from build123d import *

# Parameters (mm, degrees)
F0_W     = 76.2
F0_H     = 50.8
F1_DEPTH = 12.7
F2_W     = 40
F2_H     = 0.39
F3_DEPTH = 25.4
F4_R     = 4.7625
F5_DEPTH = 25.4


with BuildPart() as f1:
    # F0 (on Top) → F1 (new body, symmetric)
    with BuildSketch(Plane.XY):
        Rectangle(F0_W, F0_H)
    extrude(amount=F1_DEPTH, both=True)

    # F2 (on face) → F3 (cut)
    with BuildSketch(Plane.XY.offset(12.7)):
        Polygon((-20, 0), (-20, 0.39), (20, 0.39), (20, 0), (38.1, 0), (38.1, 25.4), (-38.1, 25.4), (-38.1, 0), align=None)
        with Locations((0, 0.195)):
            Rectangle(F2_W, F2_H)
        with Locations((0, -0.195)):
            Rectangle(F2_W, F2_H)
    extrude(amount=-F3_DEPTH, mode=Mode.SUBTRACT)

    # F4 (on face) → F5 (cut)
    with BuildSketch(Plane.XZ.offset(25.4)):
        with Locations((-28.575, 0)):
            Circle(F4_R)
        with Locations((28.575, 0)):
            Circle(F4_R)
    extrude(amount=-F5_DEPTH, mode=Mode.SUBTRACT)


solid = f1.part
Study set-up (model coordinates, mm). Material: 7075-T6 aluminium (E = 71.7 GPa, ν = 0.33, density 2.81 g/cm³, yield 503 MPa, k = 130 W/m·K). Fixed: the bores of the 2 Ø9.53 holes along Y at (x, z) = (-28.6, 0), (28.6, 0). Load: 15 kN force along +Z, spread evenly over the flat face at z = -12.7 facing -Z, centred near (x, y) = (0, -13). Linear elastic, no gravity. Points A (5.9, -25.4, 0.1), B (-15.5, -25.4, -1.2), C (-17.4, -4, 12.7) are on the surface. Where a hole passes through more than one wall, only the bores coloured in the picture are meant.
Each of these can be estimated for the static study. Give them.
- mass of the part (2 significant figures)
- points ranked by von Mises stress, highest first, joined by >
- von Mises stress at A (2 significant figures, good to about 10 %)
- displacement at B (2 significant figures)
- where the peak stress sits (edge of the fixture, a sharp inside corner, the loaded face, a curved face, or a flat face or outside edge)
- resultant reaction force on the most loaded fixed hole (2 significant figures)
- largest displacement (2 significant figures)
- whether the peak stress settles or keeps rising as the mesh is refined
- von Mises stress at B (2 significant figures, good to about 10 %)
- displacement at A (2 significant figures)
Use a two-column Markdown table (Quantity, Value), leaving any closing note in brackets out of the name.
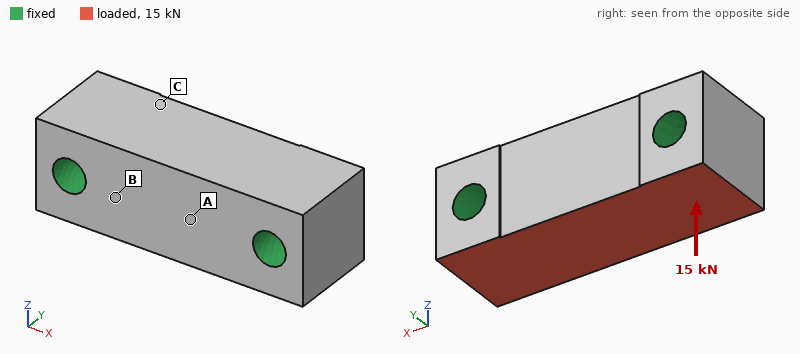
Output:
| Quantity | Value |
|---|---|
| mass of the part | 130 g |
| points ranked by von Mises stress, highest first, joined by > | B > A > C |
| von Mises stress at A | 6.3 MPa |
| displacement at B | 4.6 µm |
| where the peak stress sits | edge of the fixture |
| resultant reaction force on the most loaded fixed hole | 7.5 kN |
| largest displacement | 8.6 µm |
| whether the peak stress settles or keeps rising as the mesh is refined | keeps rising |
| von Mises stress at B | 13 MPa |
| displacement at A | 7.3 µm |
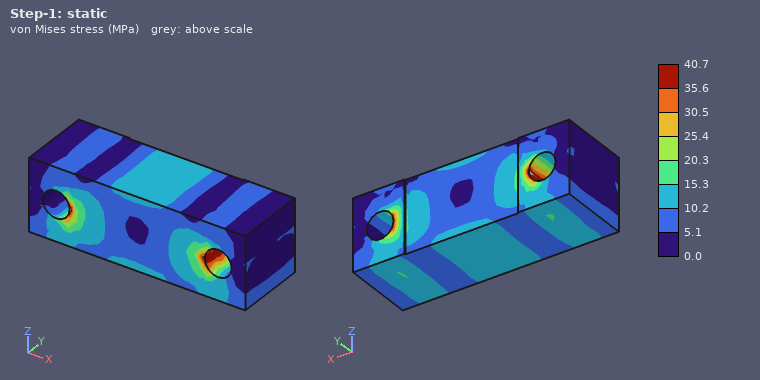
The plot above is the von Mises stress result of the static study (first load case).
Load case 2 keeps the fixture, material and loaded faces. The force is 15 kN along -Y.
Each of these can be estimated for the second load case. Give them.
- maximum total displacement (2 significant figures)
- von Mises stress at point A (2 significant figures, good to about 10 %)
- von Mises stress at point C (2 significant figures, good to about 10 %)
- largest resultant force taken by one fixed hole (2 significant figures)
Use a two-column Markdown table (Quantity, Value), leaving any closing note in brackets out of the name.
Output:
| Quantity | Value |
|---|---|
| maximum total displacement | 20 µm |
| von Mises stress at point A | 14 MPa |
| von Mises stress at point C | 7.8 MPa |
| largest resultant force taken by one fixed hole | 7.5 kN |
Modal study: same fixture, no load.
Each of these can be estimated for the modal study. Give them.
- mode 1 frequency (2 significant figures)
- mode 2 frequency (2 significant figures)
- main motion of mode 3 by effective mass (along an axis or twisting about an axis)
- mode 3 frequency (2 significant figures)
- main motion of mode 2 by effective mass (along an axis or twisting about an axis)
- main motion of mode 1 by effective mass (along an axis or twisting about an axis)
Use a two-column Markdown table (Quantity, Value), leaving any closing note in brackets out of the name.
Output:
| Quantity | Value |
|---|---|
| mode 1 frequency | 21 kHz |
| mode 2 frequency | 23 kHz |
| main motion of mode 3 by effective mass | twisting about X |
| mode 3 frequency | 27 kHz |
| main motion of mode 2 by effective mass | along Y |
| main motion of mode 1 by effective mass | along Z |
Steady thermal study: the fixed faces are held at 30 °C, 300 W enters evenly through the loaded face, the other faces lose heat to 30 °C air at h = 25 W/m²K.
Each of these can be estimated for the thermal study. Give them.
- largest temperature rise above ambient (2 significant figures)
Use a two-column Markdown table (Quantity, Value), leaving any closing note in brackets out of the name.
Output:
| Quantity | Value |
|---|---|
| largest temperature rise above ambient | 28 K |
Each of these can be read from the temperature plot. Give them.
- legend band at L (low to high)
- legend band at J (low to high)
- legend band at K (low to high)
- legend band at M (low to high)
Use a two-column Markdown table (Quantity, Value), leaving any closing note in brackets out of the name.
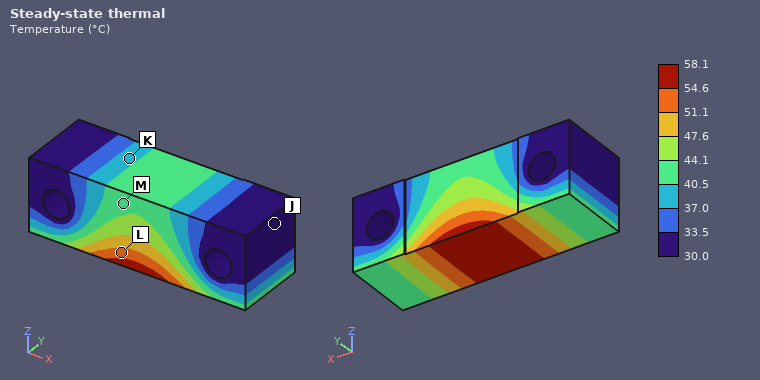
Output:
| Quantity | Value |
|---|---|
| legend band at L | 51.1 to 54.6 °C |
| legend band at J | 30.0 to 33.5 °C |
| legend band at K | 37.0 to 40.5 °C |
| legend band at M | 40.5 to 44.1 °C |
